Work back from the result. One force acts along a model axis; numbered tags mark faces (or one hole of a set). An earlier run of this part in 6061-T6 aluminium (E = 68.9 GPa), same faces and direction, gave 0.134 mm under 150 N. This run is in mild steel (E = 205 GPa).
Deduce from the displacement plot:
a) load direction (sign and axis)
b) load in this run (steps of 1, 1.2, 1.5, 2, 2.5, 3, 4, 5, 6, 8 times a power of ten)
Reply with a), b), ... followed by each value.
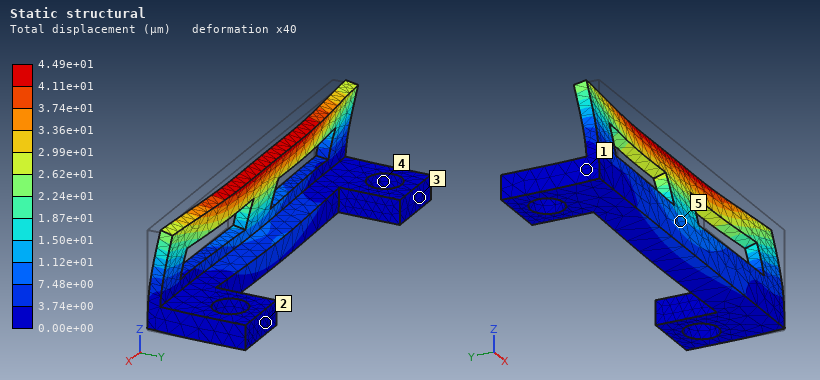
a) +Y
b) 150 N
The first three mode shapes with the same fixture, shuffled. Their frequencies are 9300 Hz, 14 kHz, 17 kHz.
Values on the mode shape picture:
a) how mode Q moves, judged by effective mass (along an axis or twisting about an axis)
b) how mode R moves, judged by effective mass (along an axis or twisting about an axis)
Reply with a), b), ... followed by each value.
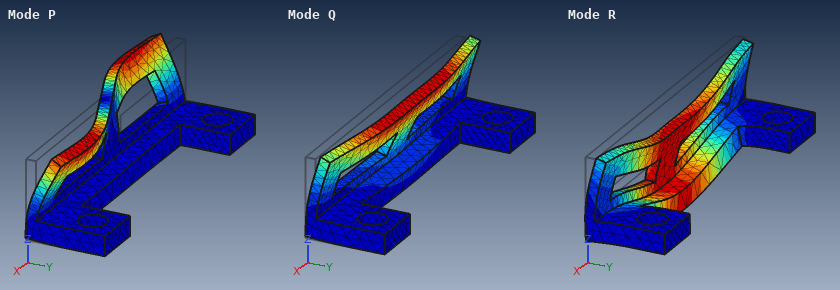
a) along Y
b) along Z
